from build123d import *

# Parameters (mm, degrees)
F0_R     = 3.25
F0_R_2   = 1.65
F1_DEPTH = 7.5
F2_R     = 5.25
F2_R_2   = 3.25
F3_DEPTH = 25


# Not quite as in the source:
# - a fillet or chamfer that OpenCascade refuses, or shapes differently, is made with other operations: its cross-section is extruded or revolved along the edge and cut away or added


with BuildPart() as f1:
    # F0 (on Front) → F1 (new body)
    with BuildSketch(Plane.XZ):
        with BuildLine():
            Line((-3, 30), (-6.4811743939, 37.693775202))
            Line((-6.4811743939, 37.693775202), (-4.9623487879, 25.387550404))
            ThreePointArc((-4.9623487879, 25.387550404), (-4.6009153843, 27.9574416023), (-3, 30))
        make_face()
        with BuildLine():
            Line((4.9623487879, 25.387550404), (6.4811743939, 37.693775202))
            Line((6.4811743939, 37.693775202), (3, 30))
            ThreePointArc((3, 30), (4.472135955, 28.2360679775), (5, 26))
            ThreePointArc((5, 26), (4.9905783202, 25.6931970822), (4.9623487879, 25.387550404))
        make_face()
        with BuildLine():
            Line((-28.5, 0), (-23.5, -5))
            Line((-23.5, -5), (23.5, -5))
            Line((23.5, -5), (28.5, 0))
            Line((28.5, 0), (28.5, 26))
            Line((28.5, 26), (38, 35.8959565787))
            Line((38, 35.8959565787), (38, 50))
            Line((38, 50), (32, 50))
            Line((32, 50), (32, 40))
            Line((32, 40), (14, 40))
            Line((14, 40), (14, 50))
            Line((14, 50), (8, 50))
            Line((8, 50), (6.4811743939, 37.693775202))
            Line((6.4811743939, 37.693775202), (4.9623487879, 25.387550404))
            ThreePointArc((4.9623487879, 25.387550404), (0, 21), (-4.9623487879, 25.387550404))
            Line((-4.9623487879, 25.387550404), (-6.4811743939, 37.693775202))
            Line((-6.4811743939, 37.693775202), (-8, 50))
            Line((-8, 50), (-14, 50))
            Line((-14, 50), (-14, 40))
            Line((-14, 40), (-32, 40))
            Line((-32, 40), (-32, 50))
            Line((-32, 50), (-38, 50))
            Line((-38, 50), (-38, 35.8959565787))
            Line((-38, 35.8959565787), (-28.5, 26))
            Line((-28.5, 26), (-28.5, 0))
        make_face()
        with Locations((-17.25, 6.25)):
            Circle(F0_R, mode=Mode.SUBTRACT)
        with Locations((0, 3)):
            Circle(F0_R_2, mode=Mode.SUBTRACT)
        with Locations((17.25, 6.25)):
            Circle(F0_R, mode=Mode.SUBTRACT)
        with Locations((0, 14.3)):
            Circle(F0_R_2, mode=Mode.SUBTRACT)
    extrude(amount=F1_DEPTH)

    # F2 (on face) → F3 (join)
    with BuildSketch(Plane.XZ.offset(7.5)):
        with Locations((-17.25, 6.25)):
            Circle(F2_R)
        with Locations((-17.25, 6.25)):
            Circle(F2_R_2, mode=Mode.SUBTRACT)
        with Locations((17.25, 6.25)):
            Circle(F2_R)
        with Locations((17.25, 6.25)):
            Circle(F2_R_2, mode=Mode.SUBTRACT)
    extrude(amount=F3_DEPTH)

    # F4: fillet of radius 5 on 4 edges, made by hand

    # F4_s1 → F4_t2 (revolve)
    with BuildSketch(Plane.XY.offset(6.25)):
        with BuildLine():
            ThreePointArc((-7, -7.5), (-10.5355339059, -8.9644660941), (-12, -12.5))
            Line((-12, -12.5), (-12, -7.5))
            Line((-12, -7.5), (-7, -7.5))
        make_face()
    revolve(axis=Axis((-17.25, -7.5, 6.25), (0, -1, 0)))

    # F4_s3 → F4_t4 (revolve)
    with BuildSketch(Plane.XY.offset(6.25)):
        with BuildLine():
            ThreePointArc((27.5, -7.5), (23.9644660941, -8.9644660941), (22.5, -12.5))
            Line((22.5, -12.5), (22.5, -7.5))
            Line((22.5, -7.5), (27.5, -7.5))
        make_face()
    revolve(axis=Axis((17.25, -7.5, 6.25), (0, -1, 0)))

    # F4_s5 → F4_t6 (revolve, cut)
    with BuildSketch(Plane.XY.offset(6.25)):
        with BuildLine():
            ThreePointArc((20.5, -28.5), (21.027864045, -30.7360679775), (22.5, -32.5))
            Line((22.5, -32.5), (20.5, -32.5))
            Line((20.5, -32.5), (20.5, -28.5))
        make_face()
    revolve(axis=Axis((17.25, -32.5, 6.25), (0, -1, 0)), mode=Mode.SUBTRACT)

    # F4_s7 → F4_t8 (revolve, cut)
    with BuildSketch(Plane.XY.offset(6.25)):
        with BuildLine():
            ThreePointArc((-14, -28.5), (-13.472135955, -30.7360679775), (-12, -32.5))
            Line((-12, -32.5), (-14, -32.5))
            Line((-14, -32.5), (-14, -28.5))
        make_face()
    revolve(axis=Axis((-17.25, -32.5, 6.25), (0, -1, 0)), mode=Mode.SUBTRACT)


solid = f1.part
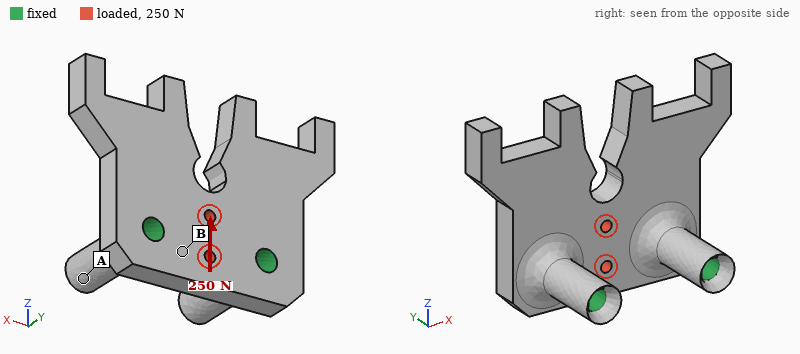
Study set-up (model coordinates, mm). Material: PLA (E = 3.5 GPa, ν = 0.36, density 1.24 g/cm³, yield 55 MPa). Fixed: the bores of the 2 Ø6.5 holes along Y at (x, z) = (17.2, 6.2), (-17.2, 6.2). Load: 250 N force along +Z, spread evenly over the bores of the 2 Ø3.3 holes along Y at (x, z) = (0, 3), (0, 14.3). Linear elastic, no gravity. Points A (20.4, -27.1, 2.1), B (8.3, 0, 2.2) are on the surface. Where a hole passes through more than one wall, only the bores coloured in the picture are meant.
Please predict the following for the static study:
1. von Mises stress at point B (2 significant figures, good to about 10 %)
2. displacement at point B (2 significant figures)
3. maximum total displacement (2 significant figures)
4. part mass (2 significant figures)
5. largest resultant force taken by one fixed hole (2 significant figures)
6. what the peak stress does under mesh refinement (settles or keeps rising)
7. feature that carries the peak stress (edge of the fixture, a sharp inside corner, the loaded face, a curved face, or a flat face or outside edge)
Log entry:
1.3 MPa
6.1 µm
18 µm
29 g
130 N
keeps rising
edge of the fixture
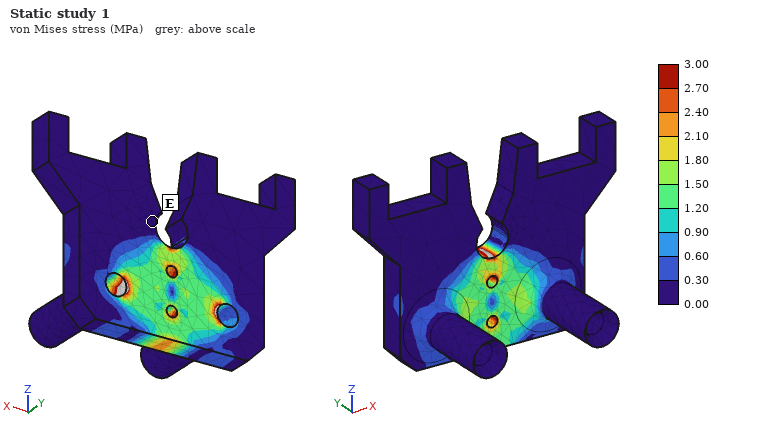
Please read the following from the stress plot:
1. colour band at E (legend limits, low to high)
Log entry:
0.00 to 0.30 MPa
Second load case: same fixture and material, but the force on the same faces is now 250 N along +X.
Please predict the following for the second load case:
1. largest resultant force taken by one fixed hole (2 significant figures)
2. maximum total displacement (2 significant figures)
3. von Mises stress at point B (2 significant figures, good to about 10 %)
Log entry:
130 N
6.1 µm
0.82 MPa
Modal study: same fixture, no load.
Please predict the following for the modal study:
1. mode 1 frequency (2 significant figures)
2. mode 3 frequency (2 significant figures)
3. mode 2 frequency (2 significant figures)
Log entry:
1400 Hz
2700 Hz
1400 Hz
